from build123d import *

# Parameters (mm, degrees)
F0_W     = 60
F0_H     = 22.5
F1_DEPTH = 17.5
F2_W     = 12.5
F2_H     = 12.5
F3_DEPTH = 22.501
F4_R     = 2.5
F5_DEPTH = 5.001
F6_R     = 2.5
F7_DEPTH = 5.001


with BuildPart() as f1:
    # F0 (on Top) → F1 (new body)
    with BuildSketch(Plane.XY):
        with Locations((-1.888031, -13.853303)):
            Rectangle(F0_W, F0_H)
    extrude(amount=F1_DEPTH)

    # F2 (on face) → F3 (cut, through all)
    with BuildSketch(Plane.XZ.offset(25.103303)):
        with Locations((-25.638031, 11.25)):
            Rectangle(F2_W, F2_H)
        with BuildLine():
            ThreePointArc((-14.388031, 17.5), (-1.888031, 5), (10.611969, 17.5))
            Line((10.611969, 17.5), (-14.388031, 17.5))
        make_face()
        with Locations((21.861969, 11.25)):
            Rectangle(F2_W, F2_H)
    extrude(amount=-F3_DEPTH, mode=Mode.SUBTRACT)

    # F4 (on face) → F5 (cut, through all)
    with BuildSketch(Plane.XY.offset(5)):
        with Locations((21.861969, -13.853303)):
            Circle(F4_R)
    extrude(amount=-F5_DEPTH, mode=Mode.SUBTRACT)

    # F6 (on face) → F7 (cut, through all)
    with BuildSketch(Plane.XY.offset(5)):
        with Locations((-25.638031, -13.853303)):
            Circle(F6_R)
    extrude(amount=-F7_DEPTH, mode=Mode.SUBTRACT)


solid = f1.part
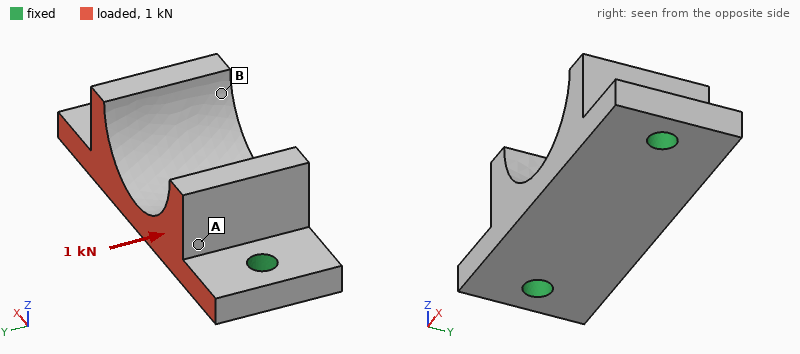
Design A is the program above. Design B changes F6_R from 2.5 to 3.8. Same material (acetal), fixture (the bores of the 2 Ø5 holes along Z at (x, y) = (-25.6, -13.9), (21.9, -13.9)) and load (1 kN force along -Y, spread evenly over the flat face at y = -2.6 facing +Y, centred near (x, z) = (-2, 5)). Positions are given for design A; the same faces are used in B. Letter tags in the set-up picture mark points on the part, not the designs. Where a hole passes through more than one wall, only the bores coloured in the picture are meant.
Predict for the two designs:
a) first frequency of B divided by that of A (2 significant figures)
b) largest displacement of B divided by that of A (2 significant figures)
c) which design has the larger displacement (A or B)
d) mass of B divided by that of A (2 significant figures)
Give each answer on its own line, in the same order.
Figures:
1.1
0.89
A
0.99
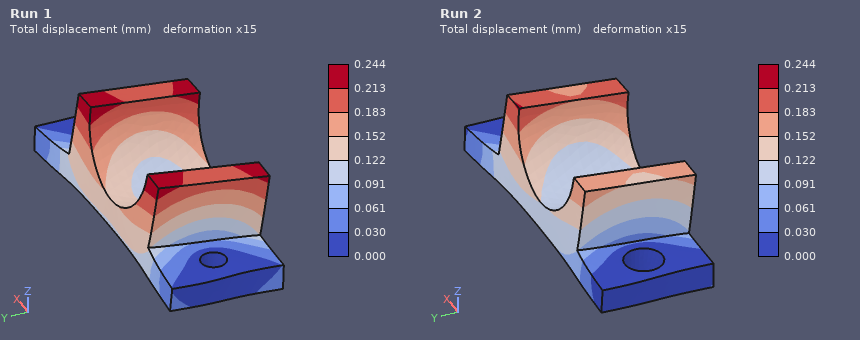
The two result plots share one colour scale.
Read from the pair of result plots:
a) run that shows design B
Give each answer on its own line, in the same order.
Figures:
Run 2
